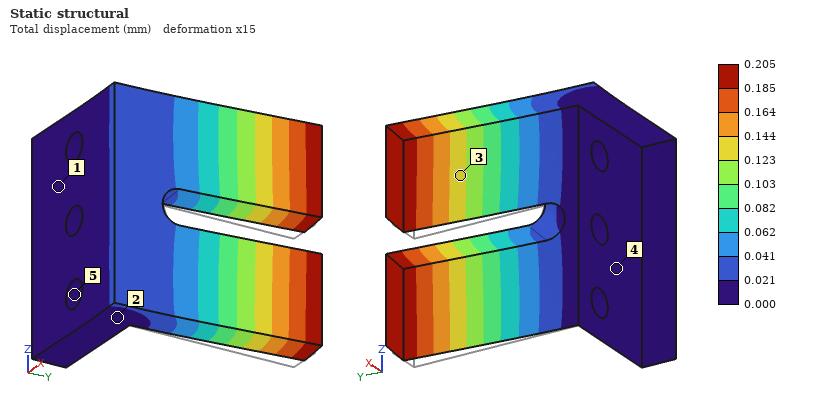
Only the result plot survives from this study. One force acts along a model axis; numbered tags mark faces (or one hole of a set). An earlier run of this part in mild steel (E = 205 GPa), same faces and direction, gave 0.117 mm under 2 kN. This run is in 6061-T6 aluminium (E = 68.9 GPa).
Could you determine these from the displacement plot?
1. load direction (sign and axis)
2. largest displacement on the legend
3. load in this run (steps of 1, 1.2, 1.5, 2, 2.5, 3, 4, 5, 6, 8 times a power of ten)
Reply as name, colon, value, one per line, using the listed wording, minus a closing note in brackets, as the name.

load direction: +X
largest displacement on the legend: 0.205 mm
load in this run: 1.2 kN
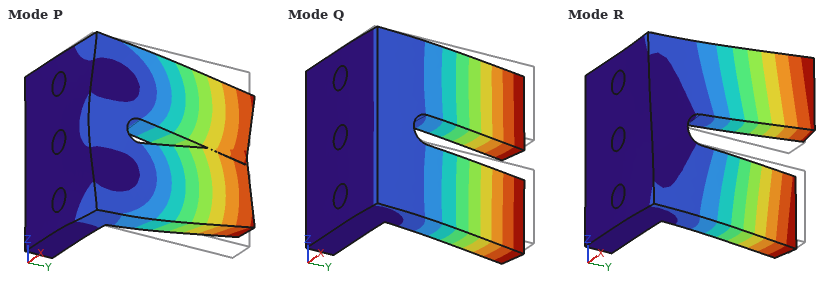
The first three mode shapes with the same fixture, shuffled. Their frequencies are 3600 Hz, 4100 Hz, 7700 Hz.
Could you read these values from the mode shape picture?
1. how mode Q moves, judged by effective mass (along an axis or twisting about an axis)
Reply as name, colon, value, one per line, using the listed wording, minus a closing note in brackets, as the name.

how mode Q moves, judged by effective mass: along X
